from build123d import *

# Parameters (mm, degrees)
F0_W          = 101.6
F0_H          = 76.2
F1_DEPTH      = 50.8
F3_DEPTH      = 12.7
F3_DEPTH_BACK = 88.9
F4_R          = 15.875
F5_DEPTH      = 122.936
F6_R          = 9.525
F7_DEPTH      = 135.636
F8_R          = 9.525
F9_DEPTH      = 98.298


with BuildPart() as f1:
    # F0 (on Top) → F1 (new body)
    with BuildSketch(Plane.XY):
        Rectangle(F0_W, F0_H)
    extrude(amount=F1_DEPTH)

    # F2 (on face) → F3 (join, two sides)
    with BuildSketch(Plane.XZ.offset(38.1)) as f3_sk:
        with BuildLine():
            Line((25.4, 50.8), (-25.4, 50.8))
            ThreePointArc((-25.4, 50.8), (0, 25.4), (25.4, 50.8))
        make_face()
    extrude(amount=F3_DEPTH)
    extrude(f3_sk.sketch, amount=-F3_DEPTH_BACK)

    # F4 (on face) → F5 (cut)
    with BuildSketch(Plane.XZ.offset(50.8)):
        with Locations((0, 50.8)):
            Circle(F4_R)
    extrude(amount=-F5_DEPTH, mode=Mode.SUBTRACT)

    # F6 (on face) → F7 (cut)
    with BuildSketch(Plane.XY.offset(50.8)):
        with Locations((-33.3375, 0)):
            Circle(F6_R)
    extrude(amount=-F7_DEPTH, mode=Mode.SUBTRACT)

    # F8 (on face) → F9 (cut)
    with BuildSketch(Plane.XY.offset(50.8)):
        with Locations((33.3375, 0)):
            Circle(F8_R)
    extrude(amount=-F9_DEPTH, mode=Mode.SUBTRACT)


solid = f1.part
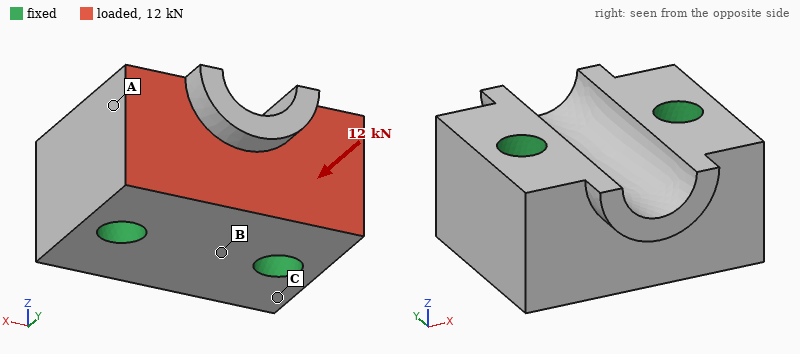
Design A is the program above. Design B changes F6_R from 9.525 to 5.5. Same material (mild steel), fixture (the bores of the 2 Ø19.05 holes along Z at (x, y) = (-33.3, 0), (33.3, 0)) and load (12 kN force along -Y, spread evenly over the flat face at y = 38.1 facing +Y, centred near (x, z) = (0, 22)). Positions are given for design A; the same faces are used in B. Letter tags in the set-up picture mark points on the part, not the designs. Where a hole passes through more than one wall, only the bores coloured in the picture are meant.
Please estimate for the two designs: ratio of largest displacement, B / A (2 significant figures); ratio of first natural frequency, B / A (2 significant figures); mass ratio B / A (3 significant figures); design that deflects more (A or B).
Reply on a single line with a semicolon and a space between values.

1.1; 0.88; 1.03; B
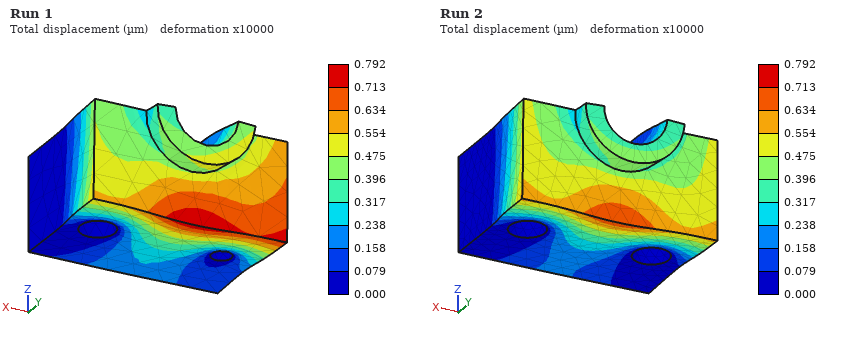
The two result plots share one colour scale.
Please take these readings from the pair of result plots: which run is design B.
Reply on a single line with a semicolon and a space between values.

Run 1
